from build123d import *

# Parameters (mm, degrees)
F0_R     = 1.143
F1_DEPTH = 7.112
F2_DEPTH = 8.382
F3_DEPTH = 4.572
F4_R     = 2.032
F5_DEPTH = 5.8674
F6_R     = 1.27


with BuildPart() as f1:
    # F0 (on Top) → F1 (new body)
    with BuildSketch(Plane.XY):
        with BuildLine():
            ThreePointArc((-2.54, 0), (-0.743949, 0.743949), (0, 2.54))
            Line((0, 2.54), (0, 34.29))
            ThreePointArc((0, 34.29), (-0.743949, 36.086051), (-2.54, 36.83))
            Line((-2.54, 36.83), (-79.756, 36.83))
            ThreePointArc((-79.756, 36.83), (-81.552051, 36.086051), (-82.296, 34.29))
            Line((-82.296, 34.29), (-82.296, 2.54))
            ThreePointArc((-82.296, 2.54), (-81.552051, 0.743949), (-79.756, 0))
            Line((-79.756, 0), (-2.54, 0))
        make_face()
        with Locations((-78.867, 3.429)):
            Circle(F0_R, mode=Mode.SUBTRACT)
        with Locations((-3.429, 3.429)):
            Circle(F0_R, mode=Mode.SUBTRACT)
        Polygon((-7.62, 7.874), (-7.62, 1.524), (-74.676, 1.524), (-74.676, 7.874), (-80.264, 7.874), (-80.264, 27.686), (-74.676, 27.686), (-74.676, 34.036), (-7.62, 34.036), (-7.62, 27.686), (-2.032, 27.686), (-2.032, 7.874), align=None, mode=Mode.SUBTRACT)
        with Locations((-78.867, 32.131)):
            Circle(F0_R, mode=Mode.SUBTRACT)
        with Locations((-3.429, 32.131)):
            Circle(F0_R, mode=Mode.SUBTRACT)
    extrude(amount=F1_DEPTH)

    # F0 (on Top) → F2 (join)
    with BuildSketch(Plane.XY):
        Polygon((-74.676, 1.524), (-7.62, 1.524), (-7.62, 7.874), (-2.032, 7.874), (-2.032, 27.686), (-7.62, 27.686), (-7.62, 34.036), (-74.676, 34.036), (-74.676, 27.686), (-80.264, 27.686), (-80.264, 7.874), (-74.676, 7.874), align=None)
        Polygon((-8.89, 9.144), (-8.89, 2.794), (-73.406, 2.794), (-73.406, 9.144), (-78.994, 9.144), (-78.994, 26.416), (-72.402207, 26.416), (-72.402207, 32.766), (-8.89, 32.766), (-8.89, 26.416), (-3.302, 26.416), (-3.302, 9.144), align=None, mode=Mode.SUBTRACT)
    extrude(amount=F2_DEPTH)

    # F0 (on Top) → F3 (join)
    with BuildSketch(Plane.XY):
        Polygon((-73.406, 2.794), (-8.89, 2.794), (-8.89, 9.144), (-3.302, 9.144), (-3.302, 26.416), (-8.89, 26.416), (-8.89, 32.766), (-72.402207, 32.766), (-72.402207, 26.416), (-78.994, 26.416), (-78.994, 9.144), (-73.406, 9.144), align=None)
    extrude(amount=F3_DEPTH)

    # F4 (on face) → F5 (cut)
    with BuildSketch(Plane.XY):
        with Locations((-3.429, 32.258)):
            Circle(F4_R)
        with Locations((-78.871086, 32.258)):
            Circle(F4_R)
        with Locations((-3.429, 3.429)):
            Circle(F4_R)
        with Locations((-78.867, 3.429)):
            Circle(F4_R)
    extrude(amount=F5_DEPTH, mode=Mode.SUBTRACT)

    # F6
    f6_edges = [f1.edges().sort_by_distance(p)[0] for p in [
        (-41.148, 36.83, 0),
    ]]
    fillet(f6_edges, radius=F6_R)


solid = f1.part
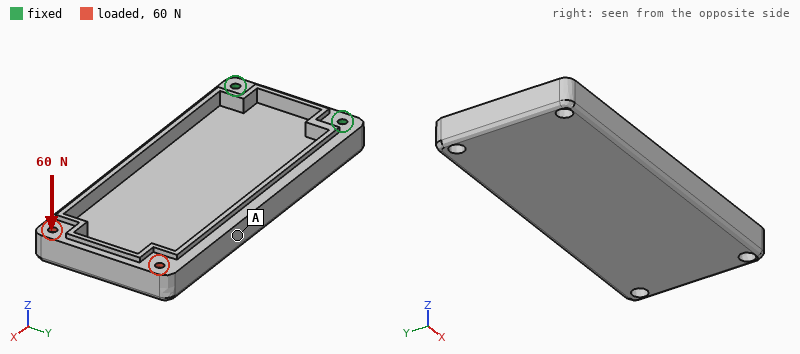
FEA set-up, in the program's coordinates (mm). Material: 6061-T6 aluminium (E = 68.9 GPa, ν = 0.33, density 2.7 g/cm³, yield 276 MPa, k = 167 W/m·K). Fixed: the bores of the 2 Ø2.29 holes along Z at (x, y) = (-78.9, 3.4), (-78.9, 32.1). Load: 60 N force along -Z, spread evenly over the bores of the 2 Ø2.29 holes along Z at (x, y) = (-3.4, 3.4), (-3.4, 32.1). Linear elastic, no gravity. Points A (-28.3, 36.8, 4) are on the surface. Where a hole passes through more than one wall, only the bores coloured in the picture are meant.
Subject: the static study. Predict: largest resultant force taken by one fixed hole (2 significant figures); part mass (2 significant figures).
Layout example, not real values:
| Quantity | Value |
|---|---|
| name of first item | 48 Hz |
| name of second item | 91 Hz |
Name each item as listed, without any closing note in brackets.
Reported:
| Quantity | Value |
|---|---|
| largest resultant force taken by one fixed hole | 46 N |
| part mass | 43 g |
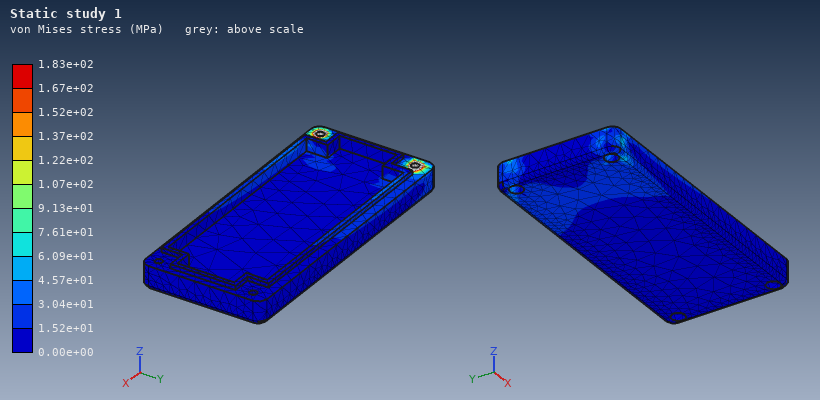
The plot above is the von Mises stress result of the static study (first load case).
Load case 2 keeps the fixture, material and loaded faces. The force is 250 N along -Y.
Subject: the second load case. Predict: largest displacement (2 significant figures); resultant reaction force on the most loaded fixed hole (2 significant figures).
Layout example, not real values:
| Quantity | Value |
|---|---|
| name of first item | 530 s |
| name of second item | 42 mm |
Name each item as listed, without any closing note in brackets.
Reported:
| Quantity | Value |
|---|---|
| largest displacement | 0.12 mm |
| resultant reaction force on the most loaded fixed hole | 650 N |
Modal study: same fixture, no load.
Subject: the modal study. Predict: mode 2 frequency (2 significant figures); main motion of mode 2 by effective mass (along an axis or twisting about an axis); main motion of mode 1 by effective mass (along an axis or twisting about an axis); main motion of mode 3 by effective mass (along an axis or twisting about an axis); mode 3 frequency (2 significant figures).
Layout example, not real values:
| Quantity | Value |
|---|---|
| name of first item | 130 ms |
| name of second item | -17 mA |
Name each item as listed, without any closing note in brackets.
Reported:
| Quantity | Value |
|---|---|
| mode 2 frequency | 2100 Hz |
| main motion of mode 2 by effective mass | along Y |
| main motion of mode 1 by effective mass | along Z |
| main motion of mode 3 by effective mass | along Y |
| mode 3 frequency | 3200 Hz |
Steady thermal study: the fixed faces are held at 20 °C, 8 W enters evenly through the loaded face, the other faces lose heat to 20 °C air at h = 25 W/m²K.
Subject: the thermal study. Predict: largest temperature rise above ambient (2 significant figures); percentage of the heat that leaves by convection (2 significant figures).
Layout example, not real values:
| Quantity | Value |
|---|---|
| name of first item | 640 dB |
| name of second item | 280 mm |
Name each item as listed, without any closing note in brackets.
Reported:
| Quantity | Value |
|---|---|
| largest temperature rise above ambient | 23 K |
| percentage of the heat that leaves by convection | 28 % |
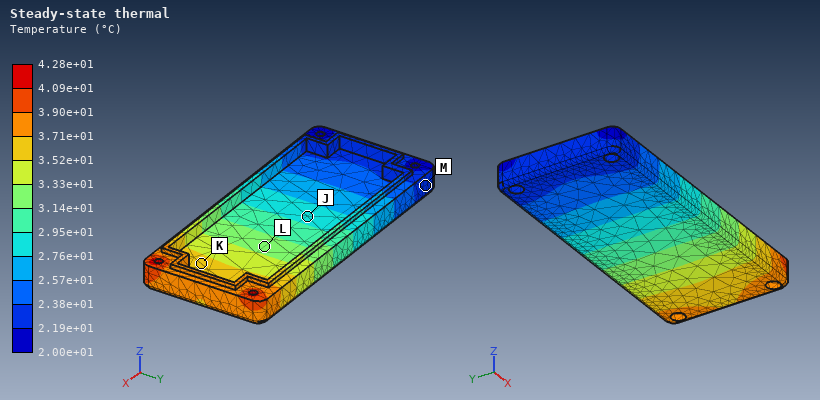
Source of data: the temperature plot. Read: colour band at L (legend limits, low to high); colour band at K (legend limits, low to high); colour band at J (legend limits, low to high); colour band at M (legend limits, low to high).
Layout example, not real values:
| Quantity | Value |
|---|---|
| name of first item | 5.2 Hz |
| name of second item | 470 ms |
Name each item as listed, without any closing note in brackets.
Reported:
| Quantity | Value |
|---|---|
| colour band at L | 3.14e+01 to 3.33e+01 °C |
| colour band at K | 3.52e+01 to 3.71e+01 °C |
| colour band at J | 2.76e+01 to 2.95e+01 °C |
| colour band at M | 2.19e+01 to 2.38e+01 °C |
